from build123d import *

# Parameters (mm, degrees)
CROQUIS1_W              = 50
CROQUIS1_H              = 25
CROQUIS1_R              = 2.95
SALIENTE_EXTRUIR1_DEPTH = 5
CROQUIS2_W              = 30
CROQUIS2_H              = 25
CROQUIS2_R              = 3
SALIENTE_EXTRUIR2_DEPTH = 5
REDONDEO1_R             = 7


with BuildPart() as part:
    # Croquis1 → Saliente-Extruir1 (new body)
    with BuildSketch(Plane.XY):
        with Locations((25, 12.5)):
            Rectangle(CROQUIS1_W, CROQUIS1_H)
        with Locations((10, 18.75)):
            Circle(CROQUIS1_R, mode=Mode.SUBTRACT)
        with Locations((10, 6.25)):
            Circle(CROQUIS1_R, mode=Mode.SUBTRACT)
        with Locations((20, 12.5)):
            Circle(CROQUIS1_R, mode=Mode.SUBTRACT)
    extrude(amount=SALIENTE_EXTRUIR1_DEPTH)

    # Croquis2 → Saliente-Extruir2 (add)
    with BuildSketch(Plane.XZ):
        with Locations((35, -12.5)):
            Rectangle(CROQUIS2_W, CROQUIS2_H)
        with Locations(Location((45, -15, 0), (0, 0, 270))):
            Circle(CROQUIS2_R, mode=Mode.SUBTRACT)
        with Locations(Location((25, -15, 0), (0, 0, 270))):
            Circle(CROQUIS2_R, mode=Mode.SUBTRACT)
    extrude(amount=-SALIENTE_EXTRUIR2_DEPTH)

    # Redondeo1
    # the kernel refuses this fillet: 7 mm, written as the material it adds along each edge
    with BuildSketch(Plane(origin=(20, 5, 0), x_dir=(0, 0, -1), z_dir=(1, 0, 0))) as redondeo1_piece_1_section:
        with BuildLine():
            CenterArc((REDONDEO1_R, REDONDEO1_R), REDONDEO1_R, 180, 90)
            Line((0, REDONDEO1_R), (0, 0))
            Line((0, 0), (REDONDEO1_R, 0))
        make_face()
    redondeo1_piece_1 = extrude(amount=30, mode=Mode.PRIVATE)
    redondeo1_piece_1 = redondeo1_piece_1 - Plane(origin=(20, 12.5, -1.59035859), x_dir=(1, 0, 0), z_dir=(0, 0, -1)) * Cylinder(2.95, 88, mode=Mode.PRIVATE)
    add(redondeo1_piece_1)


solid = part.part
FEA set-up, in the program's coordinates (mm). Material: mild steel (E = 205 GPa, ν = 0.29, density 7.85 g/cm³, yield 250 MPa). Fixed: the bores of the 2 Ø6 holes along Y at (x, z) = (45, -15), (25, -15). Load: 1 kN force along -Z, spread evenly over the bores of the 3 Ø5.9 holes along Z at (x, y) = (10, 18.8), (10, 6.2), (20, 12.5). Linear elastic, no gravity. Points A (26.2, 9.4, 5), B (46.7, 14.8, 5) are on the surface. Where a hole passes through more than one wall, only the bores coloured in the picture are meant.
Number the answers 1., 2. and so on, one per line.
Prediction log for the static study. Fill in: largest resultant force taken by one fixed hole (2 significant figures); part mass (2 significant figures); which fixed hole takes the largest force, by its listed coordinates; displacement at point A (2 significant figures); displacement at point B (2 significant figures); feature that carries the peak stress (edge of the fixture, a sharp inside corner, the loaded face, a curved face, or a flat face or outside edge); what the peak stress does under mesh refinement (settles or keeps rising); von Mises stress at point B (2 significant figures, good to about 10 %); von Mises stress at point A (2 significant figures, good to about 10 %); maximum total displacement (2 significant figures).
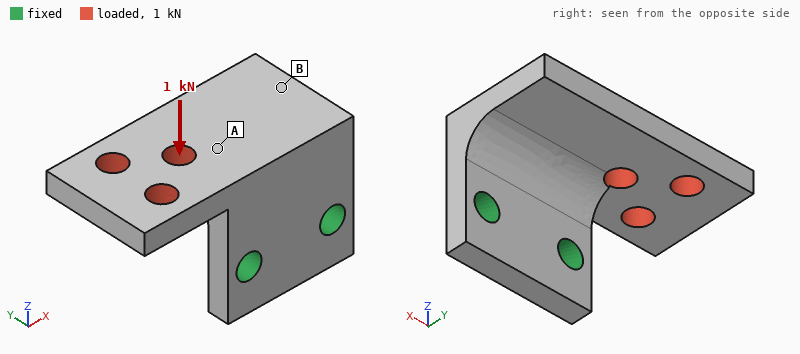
1. 1.5 kN
2. 76 g
3. (25, -15)
4. 0.031 mm
5. 0.023 mm
6. a sharp inside corner
7. keeps rising
8. 20 MPa
9. 60 MPa
10. 0.12 mm
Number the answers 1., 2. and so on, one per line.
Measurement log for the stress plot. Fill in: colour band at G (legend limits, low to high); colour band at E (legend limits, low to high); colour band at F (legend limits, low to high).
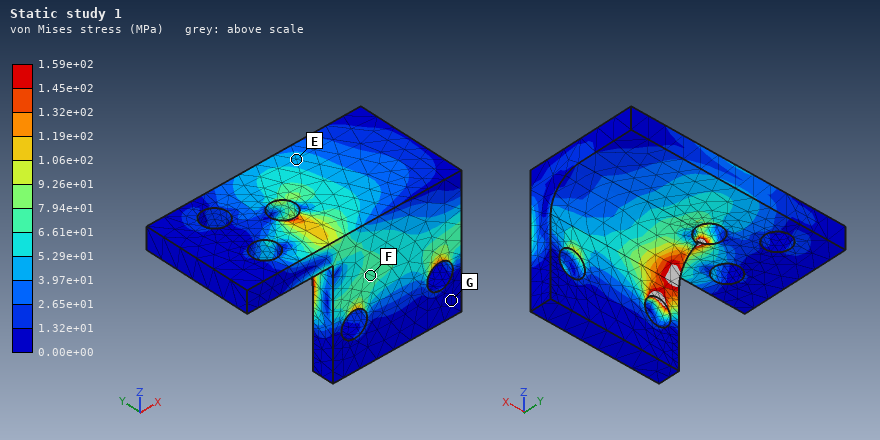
1. 0.00e+00 to 1.32e+01 MPa
2. 3.97e+01 to 5.29e+01 MPa
3. 6.61e+01 to 7.94e+01 MPa
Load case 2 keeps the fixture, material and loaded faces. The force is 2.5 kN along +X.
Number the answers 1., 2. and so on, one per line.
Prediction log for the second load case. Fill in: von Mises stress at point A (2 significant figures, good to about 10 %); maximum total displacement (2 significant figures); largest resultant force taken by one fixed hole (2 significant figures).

1. 33 MPa
2. 54 µm
3. 2.5 kN
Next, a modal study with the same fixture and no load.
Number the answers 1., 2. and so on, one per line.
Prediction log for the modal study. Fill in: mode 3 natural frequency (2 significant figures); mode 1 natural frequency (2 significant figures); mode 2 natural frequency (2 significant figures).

1. 5500 Hz
2. 3000 Hz
3. 5200 Hz
